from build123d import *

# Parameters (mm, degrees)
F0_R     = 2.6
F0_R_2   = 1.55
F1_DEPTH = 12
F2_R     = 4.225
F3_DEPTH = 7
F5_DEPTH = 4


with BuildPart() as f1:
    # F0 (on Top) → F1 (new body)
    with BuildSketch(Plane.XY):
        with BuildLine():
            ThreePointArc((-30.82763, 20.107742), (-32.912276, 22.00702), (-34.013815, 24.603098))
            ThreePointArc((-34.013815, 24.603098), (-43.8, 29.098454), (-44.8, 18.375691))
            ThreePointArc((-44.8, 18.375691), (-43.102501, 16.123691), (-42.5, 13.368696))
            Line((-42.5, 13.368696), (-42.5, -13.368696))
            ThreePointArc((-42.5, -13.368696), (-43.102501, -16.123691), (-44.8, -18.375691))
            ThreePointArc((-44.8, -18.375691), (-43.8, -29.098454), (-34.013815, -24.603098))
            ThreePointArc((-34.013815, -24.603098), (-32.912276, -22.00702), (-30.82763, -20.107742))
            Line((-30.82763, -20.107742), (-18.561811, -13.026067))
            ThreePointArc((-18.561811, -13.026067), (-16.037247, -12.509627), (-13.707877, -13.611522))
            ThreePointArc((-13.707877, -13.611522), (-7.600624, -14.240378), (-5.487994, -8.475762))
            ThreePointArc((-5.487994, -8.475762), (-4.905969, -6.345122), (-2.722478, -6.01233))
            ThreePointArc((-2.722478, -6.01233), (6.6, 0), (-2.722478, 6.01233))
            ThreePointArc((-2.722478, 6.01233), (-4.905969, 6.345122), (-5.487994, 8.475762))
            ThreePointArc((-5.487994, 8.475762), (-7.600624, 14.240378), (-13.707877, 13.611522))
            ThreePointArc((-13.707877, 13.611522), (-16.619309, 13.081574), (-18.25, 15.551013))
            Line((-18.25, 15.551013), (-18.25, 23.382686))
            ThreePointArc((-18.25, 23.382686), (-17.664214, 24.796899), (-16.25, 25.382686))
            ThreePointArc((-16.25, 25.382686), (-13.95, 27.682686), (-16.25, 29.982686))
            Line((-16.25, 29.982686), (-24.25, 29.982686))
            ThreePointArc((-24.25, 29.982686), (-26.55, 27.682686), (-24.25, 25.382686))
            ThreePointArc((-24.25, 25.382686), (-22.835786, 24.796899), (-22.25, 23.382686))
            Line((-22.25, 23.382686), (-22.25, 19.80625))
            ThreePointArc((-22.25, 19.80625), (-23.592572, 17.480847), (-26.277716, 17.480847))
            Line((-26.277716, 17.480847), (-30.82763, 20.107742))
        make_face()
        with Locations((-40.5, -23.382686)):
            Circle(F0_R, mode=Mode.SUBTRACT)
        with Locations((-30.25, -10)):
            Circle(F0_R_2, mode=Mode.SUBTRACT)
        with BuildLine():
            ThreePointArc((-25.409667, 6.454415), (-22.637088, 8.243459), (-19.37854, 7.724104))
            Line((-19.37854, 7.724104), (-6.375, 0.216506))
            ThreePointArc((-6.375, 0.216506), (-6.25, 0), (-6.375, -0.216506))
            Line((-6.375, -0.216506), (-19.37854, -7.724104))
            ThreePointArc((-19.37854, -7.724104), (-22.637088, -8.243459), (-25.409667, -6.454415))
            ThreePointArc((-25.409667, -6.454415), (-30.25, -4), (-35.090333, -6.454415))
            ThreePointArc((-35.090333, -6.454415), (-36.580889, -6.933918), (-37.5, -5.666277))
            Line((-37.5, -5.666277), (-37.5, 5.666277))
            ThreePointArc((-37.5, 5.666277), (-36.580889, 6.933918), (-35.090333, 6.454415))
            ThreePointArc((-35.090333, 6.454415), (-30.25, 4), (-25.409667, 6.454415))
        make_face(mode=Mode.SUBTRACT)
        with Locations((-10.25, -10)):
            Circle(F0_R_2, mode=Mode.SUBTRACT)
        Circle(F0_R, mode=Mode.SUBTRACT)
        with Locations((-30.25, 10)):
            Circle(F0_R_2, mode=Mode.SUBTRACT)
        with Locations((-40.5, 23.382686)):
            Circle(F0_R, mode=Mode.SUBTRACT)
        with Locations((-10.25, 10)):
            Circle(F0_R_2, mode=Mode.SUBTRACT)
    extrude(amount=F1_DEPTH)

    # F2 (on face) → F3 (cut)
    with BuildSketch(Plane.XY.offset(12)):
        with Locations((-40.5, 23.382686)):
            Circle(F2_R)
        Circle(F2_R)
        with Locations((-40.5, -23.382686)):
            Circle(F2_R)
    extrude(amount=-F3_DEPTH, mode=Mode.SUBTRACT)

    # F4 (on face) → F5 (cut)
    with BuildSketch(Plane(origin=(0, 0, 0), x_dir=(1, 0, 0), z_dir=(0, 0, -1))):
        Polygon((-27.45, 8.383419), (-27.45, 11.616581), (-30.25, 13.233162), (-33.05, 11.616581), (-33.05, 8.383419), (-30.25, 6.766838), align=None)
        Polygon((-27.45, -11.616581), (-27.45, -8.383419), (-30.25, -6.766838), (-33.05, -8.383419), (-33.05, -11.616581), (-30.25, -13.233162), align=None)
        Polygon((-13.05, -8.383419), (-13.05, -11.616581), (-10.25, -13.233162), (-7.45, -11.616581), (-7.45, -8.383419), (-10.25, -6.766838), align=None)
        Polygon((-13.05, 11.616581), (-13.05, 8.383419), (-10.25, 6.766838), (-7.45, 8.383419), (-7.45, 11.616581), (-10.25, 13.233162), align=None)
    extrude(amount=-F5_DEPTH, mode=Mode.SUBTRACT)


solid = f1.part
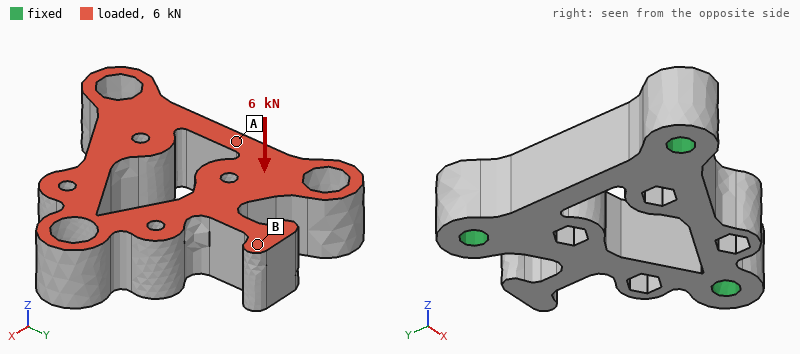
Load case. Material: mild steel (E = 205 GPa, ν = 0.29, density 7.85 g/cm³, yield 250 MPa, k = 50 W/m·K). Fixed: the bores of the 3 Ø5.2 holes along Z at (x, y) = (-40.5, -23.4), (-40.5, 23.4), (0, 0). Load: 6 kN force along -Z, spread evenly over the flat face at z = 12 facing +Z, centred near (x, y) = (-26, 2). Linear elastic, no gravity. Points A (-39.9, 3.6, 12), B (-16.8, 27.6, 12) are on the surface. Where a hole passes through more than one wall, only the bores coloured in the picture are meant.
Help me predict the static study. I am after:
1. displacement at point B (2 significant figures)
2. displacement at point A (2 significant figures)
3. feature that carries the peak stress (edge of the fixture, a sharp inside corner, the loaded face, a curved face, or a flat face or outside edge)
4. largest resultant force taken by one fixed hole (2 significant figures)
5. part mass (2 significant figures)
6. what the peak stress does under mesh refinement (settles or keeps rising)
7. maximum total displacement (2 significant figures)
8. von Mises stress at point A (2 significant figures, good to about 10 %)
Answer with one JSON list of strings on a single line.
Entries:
["18 µm", "6.0 µm", "edge of the fixture", "2.5 kN", "120 g", "keeps rising", "19 µm", "36 MPa"]
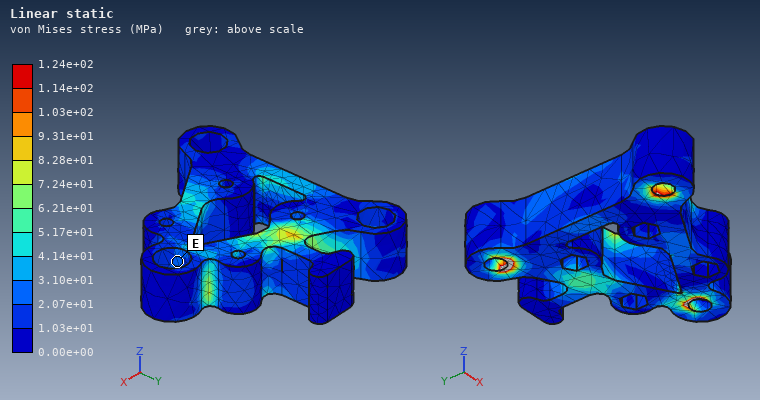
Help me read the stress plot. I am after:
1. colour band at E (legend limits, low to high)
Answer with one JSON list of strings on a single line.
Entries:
["2.07e+01 to 3.10e+01 MPa"]
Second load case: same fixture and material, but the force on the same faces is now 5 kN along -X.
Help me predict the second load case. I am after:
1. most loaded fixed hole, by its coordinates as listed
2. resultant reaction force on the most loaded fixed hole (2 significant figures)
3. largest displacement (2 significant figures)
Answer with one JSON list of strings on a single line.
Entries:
["(0, 0)", "2.4 kN", "25 µm"]
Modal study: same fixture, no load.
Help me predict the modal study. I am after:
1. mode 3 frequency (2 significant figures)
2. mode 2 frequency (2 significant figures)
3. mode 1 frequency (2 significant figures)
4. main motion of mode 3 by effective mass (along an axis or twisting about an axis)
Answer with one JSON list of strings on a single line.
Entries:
["12 kHz", "9900 Hz", "9300 Hz", "along X"]
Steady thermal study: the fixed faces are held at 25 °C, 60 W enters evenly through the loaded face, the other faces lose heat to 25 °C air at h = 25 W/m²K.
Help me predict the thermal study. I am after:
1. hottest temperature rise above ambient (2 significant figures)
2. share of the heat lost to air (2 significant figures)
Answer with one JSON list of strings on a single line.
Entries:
["61 K", "7.5 %"]
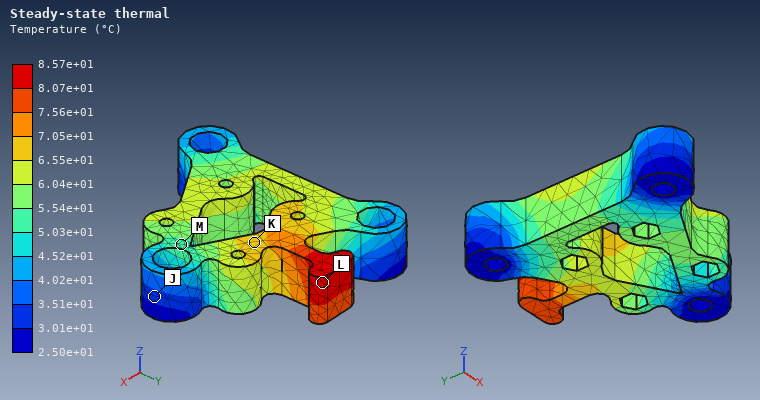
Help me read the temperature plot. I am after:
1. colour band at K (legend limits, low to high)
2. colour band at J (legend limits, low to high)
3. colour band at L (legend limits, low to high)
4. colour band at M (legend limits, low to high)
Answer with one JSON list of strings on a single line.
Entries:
["6.55e+01 to 7.05e+01 °C", "3.01e+01 to 3.51e+01 °C", "8.07e+01 to 8.57e+01 °C", "5.03e+01 to 5.54e+01 °C"]
